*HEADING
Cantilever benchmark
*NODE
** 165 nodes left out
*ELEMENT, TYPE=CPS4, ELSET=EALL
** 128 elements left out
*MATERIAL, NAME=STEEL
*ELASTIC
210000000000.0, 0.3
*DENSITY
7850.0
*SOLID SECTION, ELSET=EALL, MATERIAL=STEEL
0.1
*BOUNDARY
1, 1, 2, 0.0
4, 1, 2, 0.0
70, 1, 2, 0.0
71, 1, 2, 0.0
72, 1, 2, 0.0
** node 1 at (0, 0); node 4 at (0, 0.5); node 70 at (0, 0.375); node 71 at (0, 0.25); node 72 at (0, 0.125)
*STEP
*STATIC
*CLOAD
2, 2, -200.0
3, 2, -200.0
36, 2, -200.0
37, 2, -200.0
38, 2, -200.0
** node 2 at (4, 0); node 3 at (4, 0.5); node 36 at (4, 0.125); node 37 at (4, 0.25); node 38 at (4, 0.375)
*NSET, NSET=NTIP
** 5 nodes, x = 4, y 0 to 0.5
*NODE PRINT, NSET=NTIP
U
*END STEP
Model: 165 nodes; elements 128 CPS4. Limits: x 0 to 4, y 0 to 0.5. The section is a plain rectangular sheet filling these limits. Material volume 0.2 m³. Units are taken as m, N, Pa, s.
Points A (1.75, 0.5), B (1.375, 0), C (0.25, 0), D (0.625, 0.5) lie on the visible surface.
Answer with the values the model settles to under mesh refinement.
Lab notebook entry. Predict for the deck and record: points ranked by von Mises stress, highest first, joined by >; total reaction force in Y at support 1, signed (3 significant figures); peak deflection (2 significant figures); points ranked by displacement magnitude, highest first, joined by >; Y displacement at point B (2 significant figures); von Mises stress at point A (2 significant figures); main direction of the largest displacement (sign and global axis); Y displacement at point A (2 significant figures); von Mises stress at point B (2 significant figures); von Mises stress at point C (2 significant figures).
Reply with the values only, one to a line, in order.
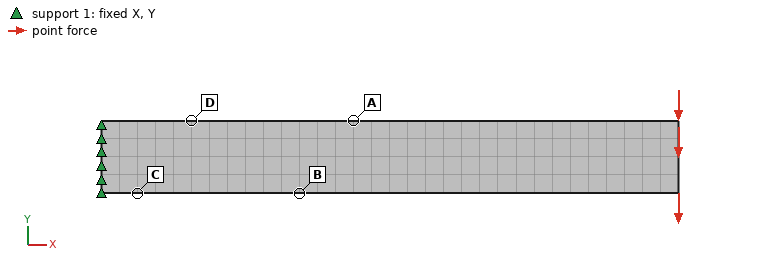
C > D > B > A
1000 N
9.9e-05 m
A > B > D > C
-1.6e-05 m
5.4e+05 Pa
-Y
-2.4e-05 m
6.3e+05 Pa
8.9e+05 Pa
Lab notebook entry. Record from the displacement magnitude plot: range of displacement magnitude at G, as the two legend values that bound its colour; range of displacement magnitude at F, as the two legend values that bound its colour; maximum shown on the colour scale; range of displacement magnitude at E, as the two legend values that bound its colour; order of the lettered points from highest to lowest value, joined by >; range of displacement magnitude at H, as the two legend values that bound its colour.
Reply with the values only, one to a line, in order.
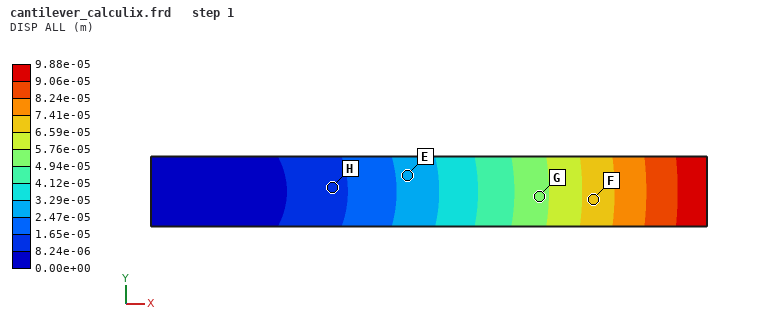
4.94e-05 to 5.76e-05 m
6.59e-05 to 7.41e-05 m
9.88e-05 m
2.47e-05 to 3.29e-05 m
F > G > E > H
8.24e-06 to 1.65e-05 m
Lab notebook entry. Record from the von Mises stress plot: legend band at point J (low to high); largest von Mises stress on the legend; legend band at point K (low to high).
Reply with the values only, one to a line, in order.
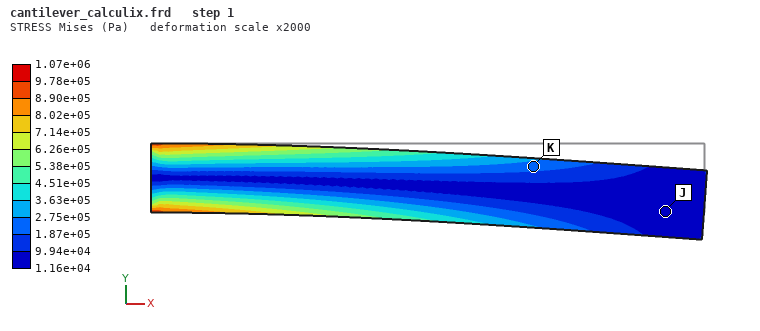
1.16e+04 to 9.94e+04 Pa
1.07e+06 Pa
1.87e+05 to 2.75e+05 Pa
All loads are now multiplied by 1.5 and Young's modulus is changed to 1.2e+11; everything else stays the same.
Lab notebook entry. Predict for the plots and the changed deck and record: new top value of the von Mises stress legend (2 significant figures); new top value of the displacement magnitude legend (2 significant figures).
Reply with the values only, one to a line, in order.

1.6e+06 Pa
2.6e-04 m
